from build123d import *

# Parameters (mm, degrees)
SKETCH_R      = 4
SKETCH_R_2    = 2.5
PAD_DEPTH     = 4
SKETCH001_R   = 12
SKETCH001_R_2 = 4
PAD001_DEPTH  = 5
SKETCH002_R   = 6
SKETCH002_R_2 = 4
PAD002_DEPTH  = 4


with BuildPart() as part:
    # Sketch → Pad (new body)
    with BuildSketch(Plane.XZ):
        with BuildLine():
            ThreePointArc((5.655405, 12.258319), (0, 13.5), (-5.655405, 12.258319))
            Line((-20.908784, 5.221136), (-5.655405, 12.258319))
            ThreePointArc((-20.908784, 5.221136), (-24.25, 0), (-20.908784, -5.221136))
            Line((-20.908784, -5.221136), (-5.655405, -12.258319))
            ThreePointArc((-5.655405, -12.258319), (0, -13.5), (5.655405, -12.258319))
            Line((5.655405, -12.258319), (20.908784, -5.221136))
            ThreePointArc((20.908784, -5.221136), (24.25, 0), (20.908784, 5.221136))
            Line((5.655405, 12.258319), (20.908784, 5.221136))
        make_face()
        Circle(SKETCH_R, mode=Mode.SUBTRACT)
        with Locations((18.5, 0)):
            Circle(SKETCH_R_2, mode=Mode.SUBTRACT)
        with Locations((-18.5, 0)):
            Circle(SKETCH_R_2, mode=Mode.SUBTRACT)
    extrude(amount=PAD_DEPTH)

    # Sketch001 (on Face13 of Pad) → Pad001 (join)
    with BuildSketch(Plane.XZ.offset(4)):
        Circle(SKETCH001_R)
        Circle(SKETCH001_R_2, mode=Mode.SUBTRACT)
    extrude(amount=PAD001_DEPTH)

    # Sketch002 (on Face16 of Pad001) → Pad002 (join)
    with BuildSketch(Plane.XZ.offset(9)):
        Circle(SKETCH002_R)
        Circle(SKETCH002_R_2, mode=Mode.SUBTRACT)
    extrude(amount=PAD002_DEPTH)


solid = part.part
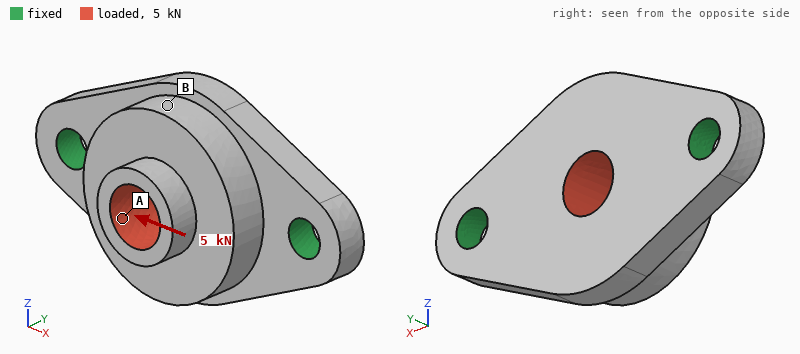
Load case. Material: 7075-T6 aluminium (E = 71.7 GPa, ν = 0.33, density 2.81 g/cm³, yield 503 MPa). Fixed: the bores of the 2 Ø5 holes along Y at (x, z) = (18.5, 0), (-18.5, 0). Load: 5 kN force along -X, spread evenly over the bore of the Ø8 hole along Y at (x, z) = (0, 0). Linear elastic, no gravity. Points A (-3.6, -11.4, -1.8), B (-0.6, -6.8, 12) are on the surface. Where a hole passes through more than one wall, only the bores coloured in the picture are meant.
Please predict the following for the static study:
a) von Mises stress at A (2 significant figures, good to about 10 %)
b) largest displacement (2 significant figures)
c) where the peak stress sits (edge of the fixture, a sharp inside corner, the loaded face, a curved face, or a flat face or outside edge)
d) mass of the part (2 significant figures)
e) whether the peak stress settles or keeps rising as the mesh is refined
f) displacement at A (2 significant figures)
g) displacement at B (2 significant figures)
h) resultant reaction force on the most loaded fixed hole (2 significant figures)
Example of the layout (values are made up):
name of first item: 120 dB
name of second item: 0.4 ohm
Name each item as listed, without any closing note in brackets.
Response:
von Mises stress at A: 38 MPa
largest displacement: 21 µm
where the peak stress sits: edge of the fixture
mass of the part: 15 g
whether the peak stress settles or keeps rising as the mesh is refined: keeps rising
displacement at A: 18 µm
displacement at B: 8.4 µm
resultant reaction force on the most loaded fixed hole: 2.6 kN
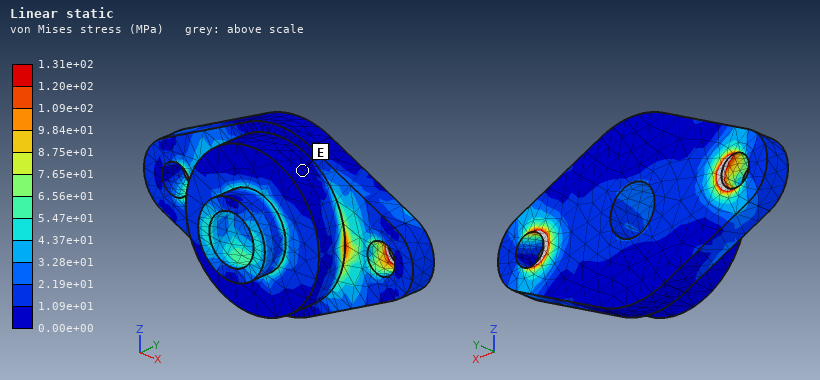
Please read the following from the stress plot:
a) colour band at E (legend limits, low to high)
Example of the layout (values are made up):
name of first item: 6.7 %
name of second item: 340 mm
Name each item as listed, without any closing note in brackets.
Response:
colour band at E: 0.00e+00 to 1.09e+01 MPa
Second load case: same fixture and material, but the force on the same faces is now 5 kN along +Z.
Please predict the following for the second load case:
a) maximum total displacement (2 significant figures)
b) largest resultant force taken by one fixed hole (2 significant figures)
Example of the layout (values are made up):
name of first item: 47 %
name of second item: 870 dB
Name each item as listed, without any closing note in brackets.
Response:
maximum total displacement: 0.13 mm
largest resultant force taken by one fixed hole: 2.5 kN
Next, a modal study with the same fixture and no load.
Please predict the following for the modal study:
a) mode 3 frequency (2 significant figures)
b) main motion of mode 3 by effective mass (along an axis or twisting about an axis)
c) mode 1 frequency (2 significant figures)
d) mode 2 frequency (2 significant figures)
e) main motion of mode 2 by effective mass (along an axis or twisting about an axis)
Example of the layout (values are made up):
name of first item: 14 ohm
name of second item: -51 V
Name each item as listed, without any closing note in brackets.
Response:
mode 3 frequency: 26 kHz
main motion of mode 3 by effective mass: along Z
mode 1 frequency: 9700 Hz
mode 2 frequency: 15 kHz
main motion of mode 2 by effective mass: along Y
